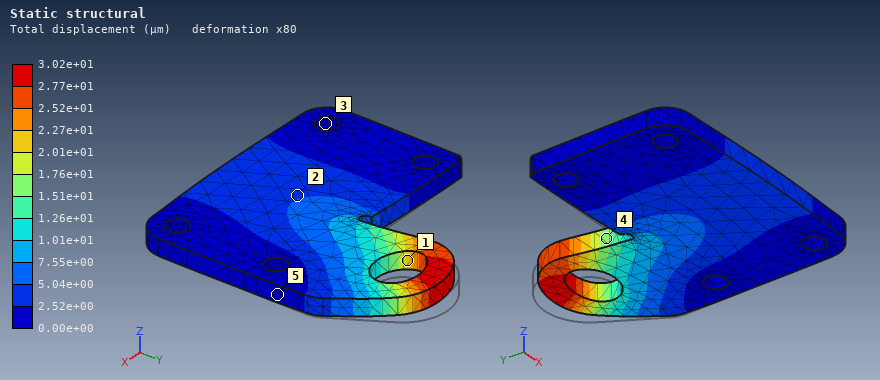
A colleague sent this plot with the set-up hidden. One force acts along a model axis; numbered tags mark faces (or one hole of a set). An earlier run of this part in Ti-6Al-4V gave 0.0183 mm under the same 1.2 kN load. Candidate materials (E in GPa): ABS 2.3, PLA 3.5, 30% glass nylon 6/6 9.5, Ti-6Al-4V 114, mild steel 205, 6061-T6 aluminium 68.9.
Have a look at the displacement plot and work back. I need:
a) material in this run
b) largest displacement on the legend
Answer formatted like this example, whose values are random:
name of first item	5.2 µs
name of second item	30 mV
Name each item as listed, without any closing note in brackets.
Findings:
material in this run	6061-T6 aluminium
largest displacement on the legend	3.02e+01 µm
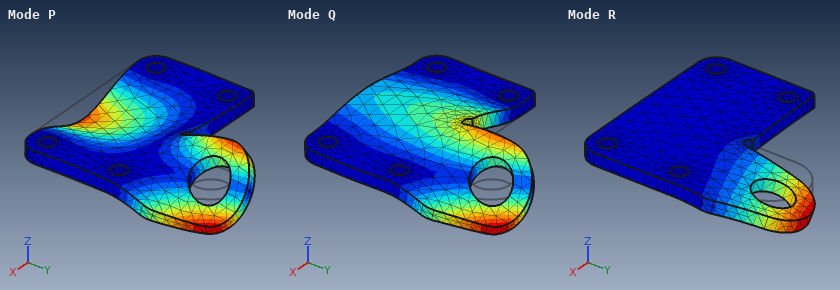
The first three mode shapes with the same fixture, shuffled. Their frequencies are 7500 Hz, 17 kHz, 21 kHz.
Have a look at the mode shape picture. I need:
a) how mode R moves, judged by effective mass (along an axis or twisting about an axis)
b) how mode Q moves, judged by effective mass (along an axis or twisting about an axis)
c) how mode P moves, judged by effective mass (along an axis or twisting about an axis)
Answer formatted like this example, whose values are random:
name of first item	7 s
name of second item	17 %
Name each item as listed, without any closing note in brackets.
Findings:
how mode R moves, judged by effective mass	along Z
how mode Q moves, judged by effective mass	along Z
how mode P moves, judged by effective mass	along Z
